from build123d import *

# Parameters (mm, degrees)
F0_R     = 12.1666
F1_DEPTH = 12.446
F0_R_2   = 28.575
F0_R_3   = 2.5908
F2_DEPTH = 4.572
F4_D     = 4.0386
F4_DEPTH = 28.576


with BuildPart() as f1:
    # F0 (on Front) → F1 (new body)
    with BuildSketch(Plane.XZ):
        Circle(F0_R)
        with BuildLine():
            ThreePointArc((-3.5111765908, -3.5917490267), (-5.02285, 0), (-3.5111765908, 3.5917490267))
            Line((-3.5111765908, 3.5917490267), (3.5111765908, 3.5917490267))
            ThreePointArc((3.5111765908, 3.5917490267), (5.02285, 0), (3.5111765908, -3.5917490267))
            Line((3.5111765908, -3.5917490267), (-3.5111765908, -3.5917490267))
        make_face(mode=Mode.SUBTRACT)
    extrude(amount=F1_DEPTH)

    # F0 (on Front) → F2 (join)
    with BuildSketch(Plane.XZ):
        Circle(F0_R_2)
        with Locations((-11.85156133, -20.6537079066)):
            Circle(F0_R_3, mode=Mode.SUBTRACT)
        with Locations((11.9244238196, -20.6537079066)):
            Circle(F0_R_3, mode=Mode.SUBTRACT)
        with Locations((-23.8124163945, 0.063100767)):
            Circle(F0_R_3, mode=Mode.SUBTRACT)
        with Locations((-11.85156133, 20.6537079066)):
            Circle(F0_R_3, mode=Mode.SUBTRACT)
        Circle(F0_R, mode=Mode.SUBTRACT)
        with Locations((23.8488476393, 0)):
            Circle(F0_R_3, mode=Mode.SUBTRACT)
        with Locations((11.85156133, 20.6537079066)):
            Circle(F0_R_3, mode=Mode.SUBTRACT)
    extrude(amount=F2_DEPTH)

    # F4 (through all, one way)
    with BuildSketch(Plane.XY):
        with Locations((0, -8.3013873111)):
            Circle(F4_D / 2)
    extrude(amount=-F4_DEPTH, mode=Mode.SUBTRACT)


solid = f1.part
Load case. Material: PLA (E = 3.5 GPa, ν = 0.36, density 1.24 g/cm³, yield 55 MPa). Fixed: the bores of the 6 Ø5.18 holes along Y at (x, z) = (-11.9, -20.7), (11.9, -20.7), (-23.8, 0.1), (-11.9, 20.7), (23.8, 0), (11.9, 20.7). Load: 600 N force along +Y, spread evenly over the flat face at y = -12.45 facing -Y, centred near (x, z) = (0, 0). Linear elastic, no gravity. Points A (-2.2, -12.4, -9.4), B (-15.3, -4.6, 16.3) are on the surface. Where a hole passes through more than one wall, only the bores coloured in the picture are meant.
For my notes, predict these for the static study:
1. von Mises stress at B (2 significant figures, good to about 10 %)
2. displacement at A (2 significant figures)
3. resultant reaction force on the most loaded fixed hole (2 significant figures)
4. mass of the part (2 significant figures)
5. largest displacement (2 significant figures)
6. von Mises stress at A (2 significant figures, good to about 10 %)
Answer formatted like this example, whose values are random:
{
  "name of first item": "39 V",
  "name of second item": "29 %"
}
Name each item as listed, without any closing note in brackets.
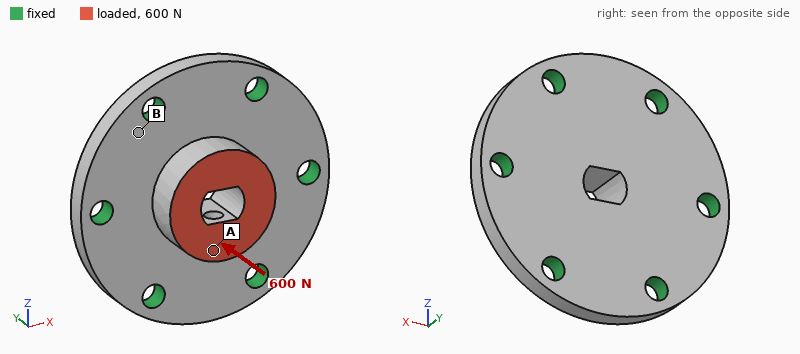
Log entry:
{
  "von Mises stress at B": "3.3 MPa",
  "displacement at A": "62 µm",
  "resultant reaction force on the most loaded fixed hole": "110 N",
  "mass of the part": "17 g",
  "largest displacement": "67 µm",
  "von Mises stress at A": "1.9 MPa"
}
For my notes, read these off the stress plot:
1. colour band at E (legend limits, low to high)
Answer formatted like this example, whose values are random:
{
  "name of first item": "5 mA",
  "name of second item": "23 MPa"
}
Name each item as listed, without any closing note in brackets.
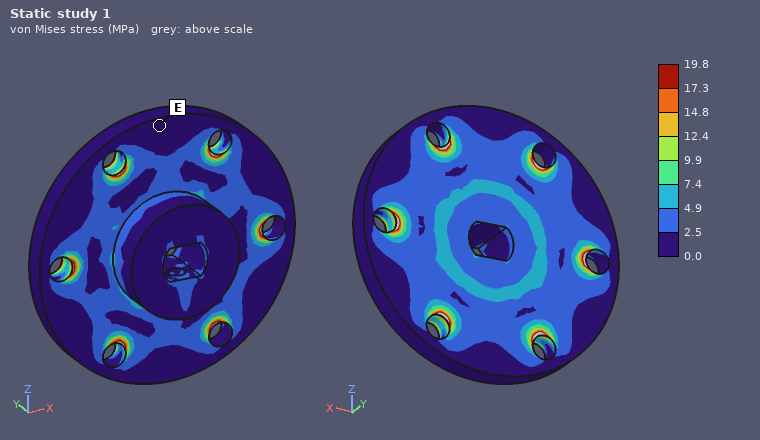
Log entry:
{
  "colour band at E": "0.0 to 2.5 MPa"
}
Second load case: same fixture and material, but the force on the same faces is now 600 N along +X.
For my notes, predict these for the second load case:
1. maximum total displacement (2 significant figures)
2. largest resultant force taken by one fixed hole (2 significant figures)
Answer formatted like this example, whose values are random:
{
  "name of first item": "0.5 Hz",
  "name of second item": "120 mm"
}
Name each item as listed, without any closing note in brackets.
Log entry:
{
  "maximum total displacement": "74 µm",
  "largest resultant force taken by one fixed hole": "190 N"
}
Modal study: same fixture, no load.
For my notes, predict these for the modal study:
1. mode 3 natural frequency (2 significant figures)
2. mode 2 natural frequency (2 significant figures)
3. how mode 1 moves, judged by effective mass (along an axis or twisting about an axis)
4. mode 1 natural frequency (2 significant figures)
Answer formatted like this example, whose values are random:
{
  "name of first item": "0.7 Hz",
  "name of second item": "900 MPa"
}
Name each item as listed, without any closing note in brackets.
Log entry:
{
  "mode 3 natural frequency": "8500 Hz",
  "mode 2 natural frequency": "8500 Hz",
  "how mode 1 moves, judged by effective mass": "along Y",
  "mode 1 natural frequency": "5800 Hz"
}
